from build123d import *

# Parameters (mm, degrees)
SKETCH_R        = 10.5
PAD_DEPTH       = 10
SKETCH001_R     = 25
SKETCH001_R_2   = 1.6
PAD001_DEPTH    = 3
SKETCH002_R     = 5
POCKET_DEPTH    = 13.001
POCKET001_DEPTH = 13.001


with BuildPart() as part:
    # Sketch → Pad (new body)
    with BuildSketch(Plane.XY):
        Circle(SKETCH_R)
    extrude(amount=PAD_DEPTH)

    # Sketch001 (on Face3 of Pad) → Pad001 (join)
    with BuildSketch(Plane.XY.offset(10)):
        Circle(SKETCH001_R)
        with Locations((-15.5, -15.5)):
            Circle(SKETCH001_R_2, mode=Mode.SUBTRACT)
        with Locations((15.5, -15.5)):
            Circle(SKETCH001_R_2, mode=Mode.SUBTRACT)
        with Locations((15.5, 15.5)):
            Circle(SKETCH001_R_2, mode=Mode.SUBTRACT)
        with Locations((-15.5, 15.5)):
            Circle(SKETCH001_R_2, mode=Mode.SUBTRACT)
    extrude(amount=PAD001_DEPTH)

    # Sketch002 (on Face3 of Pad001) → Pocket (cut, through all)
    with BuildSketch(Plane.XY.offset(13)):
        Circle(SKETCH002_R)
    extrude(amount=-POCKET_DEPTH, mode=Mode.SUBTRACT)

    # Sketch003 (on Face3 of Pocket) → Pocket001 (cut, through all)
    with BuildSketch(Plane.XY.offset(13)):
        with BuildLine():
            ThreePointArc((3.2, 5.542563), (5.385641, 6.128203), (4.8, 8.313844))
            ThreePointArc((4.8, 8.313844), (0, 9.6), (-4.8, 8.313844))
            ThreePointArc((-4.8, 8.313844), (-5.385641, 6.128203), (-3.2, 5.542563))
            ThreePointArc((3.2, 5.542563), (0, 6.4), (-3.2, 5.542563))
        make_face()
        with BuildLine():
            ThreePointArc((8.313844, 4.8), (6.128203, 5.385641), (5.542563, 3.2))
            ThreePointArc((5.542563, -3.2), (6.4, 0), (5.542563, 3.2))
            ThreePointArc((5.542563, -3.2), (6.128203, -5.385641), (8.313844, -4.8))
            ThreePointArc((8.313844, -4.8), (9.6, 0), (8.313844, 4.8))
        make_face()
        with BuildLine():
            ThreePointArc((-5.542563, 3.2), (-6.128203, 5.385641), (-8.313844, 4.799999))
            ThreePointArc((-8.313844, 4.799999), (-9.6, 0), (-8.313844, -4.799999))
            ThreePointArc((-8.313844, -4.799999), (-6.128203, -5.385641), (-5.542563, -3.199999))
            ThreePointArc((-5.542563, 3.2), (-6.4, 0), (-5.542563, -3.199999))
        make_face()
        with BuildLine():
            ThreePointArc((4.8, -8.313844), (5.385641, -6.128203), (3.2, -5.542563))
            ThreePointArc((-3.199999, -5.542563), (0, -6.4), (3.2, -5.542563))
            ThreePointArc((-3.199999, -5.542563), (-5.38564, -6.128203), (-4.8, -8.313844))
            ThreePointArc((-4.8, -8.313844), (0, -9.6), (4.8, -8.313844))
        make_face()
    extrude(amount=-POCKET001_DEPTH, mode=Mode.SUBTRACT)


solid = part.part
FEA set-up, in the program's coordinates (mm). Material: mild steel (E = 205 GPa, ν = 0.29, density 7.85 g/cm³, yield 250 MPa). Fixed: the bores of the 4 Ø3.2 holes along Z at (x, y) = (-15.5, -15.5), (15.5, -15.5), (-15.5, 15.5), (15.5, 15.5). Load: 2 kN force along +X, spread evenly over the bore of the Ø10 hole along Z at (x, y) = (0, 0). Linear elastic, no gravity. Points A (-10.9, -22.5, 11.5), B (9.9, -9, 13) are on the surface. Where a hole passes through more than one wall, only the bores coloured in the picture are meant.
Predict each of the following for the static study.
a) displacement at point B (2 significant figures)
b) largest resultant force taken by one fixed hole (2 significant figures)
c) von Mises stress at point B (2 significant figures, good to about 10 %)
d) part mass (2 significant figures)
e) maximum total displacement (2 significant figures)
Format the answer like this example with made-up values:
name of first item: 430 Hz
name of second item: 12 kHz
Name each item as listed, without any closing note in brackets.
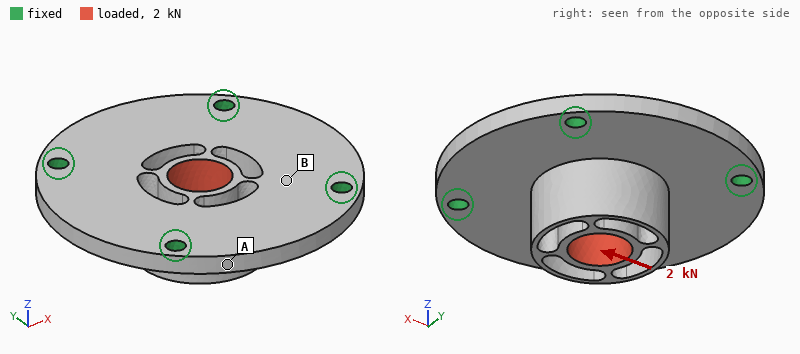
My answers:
displacement at point B: 3.9 µm
largest resultant force taken by one fixed hole: 560 N
von Mises stress at point B: 29 MPa
part mass: 50 g
maximum total displacement: 17 µm
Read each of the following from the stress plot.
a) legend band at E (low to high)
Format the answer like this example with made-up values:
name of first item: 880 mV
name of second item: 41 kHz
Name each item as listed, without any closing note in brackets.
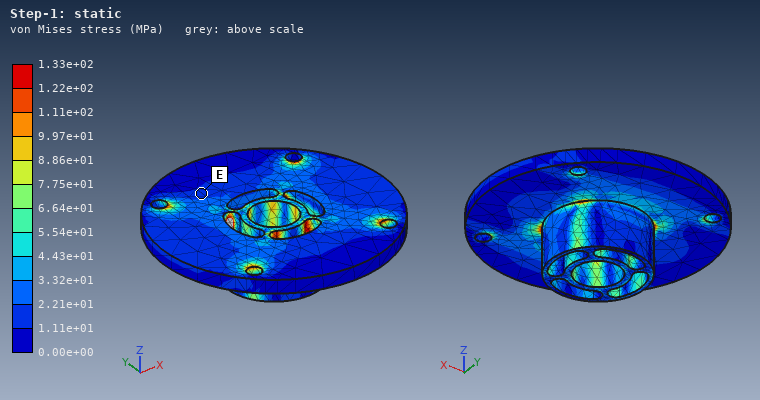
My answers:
legend band at E: 1.11e+01 to 2.21e+01 MPa
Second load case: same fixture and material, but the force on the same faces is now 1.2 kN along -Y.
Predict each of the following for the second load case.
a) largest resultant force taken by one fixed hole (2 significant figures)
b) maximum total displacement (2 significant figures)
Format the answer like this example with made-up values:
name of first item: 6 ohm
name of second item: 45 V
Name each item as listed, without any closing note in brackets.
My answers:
largest resultant force taken by one fixed hole: 340 N
maximum total displacement: 10.0 µm
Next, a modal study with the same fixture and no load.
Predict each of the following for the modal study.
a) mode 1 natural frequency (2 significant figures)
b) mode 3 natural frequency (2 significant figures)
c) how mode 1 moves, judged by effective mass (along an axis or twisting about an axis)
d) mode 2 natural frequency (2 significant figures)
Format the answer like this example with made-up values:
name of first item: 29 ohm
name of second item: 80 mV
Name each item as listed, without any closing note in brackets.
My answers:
mode 1 natural frequency: 11 kHz
mode 3 natural frequency: 14 kHz
how mode 1 moves, judged by effective mass: along Z
mode 2 natural frequency: 14 kHz
